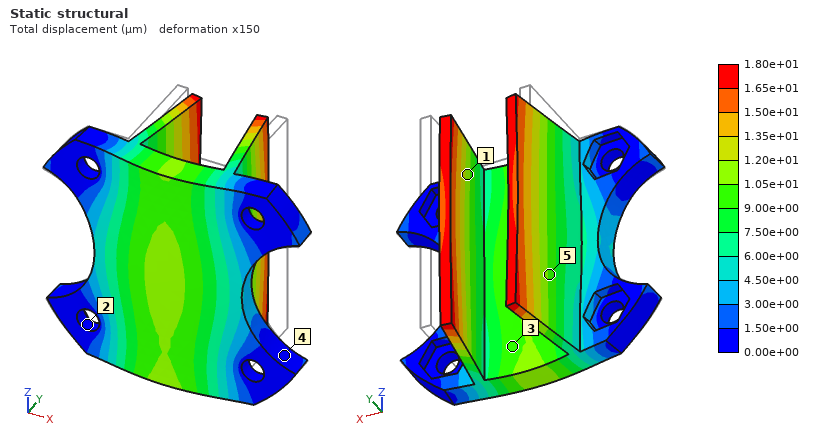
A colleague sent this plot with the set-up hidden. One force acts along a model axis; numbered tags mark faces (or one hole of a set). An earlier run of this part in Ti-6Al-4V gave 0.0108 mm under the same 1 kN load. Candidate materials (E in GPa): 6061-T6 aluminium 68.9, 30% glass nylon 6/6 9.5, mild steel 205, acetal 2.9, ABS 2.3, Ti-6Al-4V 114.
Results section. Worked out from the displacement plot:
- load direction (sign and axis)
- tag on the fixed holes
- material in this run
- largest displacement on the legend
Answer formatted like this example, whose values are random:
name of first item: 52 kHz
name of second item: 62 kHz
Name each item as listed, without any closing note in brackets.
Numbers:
load direction: -Y
tag on the fixed holes: 2
material in this run: 6061-T6 aluminium
largest displacement on the legend: 1.80e+01 µm
